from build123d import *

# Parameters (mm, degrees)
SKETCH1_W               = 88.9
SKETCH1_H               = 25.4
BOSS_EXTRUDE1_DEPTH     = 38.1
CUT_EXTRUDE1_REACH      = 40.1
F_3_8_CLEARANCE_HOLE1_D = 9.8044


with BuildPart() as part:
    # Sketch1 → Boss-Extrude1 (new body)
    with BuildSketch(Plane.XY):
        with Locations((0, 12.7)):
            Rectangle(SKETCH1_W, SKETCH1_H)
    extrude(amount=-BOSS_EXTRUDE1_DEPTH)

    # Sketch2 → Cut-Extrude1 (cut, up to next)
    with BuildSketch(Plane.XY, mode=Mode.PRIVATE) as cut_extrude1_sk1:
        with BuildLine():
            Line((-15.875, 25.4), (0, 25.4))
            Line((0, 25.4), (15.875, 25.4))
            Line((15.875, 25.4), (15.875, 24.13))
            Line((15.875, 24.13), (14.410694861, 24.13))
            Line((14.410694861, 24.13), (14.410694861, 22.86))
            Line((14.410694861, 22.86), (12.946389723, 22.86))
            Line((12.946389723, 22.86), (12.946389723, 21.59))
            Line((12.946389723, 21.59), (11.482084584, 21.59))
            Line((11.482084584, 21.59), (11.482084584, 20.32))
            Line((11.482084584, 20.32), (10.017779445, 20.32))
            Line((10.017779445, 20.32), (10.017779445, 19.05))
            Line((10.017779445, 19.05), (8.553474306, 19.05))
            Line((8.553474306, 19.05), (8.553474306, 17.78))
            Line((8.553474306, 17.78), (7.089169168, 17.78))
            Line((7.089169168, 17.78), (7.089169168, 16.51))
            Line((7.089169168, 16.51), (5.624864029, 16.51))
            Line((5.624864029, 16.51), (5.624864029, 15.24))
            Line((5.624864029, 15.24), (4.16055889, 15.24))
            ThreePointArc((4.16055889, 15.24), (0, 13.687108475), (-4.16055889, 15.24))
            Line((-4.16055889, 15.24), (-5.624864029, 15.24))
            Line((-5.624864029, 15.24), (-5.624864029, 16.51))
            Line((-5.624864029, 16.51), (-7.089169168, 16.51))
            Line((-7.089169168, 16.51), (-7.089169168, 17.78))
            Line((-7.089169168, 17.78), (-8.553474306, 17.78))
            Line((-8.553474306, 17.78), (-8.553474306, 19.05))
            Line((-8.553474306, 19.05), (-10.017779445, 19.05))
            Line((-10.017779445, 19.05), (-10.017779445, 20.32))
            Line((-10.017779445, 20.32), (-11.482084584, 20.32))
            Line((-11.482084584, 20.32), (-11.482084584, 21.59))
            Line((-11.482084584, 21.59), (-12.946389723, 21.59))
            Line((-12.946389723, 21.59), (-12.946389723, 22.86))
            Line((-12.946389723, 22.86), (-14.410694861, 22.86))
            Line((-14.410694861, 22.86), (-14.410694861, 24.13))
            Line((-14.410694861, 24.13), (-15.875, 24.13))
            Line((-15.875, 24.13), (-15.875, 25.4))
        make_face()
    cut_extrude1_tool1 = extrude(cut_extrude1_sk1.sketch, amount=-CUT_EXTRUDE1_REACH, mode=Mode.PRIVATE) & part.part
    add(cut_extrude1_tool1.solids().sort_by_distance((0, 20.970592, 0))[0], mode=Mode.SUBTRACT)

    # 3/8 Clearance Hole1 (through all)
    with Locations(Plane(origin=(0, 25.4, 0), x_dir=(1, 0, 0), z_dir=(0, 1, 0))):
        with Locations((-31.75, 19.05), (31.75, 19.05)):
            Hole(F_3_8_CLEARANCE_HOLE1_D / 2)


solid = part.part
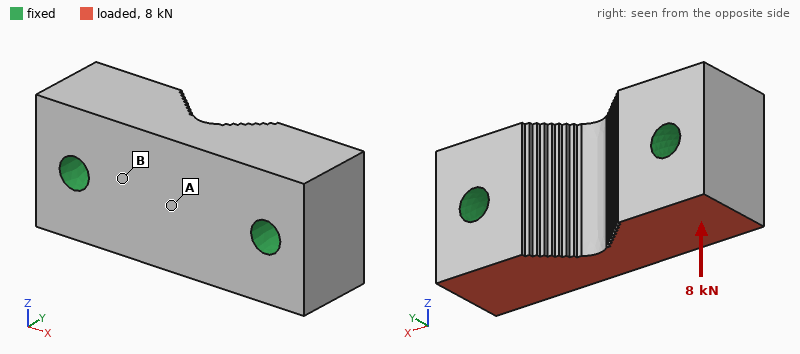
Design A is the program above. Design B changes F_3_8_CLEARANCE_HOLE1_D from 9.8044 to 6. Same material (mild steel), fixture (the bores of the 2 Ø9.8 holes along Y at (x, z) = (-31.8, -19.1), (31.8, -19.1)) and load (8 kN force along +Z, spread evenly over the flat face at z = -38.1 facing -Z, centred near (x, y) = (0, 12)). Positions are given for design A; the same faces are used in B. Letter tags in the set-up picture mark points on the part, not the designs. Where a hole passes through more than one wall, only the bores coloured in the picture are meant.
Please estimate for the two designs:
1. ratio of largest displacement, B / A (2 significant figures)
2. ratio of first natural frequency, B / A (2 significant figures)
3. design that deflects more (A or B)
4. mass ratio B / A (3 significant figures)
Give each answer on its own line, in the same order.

1.3
0.83
B
1.03
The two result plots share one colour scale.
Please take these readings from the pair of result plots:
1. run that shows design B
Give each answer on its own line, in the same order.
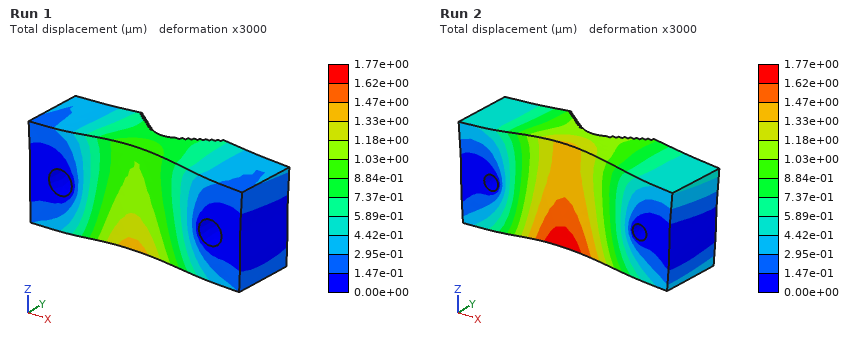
Run 2
